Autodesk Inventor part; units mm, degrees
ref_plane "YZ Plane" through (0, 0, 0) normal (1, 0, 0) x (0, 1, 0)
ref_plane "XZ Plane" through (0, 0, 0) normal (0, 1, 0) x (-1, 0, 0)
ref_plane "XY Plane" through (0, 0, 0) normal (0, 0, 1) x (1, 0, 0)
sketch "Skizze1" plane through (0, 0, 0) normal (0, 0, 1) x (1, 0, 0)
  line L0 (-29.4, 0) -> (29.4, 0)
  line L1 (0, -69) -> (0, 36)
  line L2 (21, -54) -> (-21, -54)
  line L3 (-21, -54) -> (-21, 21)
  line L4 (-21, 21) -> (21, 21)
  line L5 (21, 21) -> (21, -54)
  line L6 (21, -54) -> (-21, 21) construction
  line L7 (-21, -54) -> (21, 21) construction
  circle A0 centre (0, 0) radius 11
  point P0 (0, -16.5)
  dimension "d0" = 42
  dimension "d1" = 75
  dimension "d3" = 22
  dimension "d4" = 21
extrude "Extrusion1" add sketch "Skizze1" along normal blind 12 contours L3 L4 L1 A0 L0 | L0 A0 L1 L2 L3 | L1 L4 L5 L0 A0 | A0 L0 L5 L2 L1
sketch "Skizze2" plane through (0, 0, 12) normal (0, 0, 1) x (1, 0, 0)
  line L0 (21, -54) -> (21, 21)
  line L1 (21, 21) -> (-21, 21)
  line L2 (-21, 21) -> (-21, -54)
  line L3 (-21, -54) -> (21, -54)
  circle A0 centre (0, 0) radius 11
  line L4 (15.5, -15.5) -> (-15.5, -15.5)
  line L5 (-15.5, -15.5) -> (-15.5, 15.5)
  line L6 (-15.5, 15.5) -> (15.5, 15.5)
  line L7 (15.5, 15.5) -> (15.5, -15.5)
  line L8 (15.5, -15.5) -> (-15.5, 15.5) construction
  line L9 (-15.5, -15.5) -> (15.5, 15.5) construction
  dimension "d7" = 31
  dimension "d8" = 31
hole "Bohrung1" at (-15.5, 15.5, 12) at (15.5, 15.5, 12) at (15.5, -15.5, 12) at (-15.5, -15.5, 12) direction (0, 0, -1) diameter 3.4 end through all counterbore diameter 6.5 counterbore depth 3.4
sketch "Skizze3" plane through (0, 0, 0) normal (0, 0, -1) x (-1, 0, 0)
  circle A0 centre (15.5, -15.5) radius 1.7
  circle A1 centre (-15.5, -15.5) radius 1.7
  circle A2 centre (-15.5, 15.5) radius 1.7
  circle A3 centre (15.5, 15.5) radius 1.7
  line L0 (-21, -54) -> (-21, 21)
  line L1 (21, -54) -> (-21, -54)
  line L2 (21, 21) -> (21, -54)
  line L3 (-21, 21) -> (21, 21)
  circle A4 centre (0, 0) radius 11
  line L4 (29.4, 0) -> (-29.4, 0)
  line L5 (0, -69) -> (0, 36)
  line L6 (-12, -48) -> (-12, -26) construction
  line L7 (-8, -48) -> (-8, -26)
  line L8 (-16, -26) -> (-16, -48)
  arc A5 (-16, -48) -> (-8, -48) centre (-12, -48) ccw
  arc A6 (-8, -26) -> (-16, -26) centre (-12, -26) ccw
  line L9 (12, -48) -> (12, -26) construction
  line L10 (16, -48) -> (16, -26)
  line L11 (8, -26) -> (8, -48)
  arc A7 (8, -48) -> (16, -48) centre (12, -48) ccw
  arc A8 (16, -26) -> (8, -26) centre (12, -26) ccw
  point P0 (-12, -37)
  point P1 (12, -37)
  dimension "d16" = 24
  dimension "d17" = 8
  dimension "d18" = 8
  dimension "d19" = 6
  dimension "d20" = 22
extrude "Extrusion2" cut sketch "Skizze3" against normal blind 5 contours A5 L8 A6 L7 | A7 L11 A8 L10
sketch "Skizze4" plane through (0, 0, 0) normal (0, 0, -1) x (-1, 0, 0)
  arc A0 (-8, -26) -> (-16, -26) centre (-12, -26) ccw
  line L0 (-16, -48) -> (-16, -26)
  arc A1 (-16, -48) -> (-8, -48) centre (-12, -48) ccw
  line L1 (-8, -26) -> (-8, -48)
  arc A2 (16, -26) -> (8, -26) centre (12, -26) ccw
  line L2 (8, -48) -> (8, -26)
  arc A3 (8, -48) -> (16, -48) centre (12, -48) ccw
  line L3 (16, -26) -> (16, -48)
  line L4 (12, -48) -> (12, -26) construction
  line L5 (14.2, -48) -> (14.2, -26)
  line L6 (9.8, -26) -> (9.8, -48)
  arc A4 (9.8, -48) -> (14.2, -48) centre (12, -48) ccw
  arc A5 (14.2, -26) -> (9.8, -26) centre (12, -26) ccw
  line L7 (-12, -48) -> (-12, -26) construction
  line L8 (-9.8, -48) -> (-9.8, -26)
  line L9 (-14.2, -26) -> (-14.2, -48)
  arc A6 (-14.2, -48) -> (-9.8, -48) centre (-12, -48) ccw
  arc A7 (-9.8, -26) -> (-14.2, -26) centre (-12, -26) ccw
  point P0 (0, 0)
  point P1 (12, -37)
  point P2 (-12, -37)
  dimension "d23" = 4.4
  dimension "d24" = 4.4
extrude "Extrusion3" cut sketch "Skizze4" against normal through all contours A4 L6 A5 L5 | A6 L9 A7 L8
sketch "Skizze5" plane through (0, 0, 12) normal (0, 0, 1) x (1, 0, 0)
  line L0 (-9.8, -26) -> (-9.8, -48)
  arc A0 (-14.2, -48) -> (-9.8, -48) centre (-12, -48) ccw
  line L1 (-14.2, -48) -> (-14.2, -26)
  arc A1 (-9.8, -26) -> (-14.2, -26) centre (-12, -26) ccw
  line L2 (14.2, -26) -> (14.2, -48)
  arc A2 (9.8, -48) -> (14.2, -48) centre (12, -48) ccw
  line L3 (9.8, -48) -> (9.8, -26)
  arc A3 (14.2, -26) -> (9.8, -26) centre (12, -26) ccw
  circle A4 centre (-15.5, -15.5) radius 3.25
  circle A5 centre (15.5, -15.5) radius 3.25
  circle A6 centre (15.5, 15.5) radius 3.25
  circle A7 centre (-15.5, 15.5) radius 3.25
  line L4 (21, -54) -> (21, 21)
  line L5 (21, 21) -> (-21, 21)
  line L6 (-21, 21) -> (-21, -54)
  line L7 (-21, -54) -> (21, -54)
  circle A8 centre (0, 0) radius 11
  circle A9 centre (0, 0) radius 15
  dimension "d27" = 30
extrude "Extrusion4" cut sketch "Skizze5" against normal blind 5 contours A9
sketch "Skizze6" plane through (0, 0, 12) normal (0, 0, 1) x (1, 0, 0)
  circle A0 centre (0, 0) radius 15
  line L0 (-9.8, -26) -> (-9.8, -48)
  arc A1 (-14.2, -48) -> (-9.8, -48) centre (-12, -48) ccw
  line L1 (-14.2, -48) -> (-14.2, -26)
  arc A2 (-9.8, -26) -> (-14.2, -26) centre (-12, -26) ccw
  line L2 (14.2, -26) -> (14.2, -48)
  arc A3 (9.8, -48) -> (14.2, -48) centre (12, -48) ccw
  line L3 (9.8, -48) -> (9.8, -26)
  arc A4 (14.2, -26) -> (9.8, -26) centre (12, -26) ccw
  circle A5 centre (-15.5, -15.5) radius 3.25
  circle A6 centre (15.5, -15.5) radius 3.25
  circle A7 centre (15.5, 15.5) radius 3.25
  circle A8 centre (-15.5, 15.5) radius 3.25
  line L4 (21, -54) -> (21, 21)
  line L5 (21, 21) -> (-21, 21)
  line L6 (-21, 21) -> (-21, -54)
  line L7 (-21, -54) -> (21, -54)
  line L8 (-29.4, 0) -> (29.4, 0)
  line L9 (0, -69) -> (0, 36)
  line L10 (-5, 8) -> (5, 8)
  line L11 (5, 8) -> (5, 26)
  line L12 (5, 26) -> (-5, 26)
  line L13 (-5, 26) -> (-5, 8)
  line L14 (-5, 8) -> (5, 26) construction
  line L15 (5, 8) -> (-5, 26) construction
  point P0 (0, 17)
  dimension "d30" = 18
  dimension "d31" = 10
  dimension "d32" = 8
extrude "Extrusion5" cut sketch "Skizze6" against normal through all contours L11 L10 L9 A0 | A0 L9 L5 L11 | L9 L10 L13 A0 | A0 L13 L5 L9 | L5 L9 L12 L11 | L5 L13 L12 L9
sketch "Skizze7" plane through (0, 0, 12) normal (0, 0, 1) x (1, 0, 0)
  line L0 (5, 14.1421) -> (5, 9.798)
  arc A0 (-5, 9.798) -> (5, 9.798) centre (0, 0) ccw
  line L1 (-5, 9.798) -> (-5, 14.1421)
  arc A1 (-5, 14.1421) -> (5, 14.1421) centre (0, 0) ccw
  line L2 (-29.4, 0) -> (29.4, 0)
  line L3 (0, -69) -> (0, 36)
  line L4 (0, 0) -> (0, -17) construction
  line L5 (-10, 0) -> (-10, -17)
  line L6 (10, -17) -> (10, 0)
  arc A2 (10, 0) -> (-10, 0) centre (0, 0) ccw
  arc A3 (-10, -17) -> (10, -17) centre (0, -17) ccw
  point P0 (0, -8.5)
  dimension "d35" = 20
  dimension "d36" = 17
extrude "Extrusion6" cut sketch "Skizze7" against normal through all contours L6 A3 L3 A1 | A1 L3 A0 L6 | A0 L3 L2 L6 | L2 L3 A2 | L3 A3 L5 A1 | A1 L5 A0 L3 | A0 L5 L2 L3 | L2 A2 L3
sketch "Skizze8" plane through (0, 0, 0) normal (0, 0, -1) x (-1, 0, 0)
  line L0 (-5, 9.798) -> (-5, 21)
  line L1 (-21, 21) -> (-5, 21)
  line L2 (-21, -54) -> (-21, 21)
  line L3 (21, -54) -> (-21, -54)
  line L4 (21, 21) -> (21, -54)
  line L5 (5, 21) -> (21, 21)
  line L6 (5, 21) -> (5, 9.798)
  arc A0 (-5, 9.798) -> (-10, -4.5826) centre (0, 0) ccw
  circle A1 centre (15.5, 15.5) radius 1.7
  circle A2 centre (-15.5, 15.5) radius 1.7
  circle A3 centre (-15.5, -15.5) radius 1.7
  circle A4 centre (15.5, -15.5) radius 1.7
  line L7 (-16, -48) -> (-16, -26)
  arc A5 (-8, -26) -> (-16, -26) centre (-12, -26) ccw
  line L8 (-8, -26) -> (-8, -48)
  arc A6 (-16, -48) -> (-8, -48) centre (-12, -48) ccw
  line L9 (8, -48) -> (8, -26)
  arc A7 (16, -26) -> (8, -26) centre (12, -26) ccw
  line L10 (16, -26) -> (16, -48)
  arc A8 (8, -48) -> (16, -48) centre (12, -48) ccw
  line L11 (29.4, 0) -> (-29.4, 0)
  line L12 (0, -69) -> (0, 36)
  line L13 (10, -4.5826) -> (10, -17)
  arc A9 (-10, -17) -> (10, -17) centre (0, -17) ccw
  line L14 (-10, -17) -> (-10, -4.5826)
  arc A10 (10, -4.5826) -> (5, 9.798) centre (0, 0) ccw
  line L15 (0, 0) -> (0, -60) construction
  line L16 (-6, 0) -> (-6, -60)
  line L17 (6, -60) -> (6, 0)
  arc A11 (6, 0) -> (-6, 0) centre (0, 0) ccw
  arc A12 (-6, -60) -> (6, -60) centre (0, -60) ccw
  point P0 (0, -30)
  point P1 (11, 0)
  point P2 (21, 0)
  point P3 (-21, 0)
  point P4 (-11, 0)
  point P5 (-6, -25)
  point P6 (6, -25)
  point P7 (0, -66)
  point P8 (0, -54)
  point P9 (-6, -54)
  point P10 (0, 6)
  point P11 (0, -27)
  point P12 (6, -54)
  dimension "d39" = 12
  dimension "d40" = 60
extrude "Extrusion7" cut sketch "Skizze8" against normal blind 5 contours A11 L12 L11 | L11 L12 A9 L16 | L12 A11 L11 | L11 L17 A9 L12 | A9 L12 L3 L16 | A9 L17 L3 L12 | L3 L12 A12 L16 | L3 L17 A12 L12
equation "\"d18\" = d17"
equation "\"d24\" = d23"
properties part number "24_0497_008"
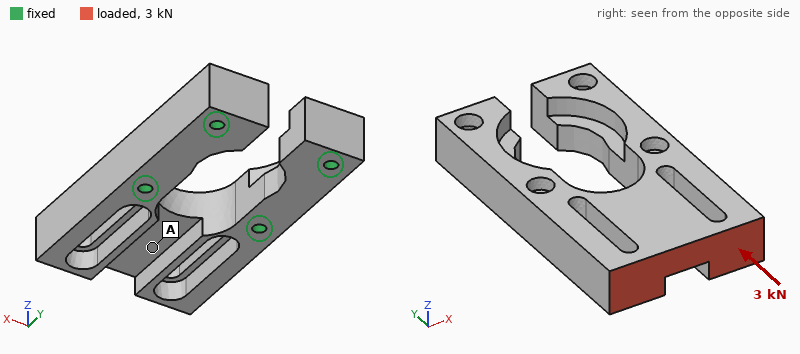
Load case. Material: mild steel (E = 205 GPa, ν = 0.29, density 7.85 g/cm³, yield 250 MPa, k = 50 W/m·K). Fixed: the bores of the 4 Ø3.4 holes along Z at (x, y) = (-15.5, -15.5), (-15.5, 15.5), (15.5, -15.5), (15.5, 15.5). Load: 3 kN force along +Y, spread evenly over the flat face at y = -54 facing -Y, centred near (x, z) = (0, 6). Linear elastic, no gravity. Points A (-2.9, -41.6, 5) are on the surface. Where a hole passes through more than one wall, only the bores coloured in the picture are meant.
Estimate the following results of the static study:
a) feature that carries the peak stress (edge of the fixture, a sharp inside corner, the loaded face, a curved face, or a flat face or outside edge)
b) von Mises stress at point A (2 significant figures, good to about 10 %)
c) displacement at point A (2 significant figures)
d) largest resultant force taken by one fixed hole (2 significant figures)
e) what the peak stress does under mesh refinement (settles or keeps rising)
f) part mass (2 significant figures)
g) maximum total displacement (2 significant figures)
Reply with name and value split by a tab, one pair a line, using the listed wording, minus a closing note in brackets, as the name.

feature that carries the peak stress	edge of the fixture
von Mises stress at point A	9.8 MPa
displacement at point A	3.2 µm
largest resultant force taken by one fixed hole	1.4 kN
what the peak stress does under mesh refinement	keeps rising
part mass	160 g
maximum total displacement	4.3 µm
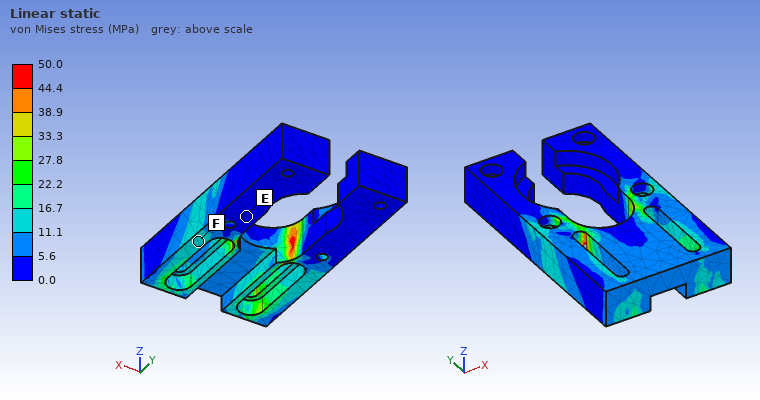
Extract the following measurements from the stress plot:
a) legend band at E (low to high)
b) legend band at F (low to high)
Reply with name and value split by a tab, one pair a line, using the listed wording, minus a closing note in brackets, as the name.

legend band at E	0.0 to 5.6 MPa
legend band at F	11.1 to 16.7 MPa
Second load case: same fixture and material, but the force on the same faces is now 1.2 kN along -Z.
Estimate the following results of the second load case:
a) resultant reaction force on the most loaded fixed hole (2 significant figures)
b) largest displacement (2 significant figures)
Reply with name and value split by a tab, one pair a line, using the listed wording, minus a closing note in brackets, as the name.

resultant reaction force on the most loaded fixed hole	850 N
largest displacement	66 µm
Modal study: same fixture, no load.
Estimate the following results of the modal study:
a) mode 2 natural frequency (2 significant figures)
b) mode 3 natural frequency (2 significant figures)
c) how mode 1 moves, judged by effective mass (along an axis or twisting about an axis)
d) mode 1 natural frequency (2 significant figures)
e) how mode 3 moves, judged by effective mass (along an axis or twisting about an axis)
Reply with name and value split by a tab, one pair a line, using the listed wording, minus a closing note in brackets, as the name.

mode 2 natural frequency	7100 Hz
mode 3 natural frequency	9500 Hz
how mode 1 moves, judged by effective mass	along Z
mode 1 natural frequency	4200 Hz
how mode 3 moves, judged by effective mass	along X
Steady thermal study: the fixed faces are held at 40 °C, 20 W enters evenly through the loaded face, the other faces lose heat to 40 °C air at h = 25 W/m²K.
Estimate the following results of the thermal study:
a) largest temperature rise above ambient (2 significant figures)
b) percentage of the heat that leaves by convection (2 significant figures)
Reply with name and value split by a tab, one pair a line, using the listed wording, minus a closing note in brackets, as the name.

largest temperature rise above ambient	54 K
percentage of the heat that leaves by convection	20 %
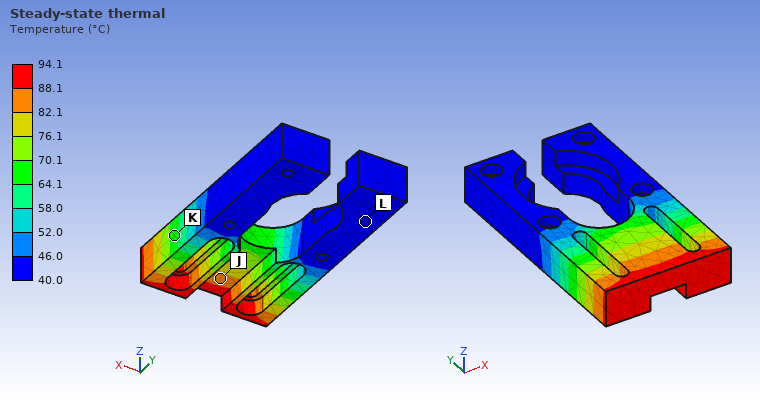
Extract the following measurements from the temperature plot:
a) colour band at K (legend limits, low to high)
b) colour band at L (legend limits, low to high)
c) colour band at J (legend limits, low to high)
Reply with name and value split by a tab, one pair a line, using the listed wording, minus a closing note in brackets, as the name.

colour band at K	64.1 to 70.1 °C
colour band at L	40.0 to 46.0 °C
colour band at J	82.1 to 88.1 °C
